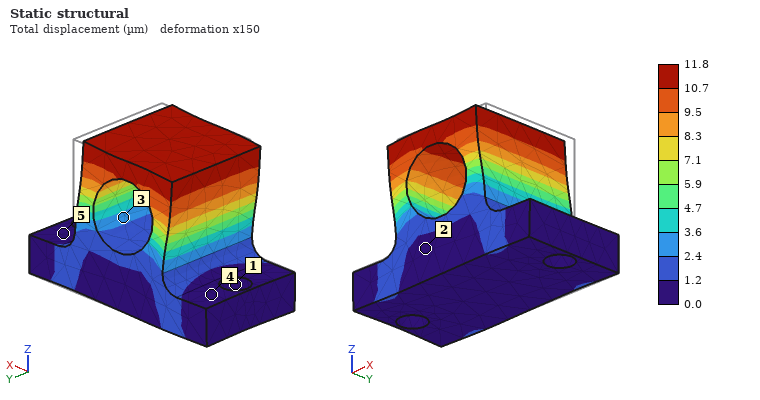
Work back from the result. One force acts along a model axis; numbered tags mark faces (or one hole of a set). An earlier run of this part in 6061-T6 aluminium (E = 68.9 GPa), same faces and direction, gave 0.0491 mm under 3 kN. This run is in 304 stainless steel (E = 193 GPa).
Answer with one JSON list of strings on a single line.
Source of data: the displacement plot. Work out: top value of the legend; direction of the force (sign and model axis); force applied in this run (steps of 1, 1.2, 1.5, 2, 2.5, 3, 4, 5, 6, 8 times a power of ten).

["11.8 µm", "-X", "2 kN"]
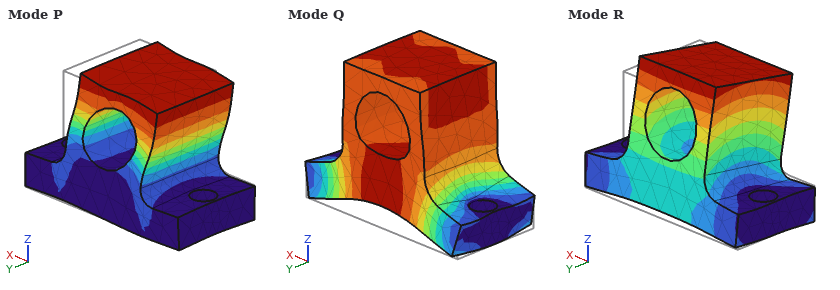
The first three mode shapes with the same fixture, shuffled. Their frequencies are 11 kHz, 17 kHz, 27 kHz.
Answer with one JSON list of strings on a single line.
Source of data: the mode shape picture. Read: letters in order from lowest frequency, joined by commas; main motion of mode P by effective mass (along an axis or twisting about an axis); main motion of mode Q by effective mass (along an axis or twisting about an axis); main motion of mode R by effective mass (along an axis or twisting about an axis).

["R, P, Q", "along X", "along Z", "along Y"]
